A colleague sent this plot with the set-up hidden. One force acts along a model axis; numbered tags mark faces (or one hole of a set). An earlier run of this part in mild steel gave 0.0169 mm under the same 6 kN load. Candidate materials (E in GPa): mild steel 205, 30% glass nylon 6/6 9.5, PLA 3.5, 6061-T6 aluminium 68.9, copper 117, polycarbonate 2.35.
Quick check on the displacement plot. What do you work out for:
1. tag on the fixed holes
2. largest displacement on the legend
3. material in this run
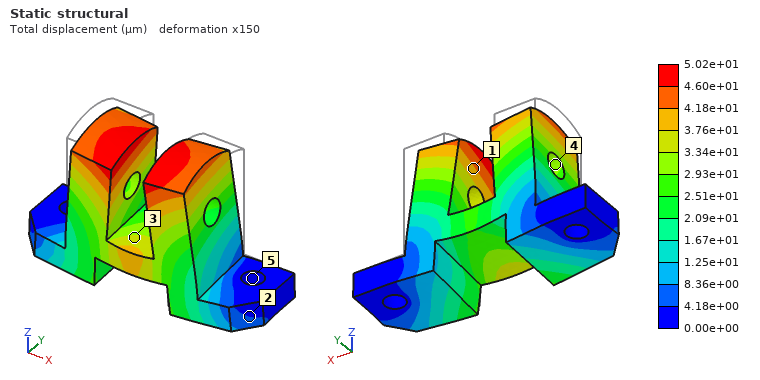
5
5.02e+01 µm
6061-T6 aluminium
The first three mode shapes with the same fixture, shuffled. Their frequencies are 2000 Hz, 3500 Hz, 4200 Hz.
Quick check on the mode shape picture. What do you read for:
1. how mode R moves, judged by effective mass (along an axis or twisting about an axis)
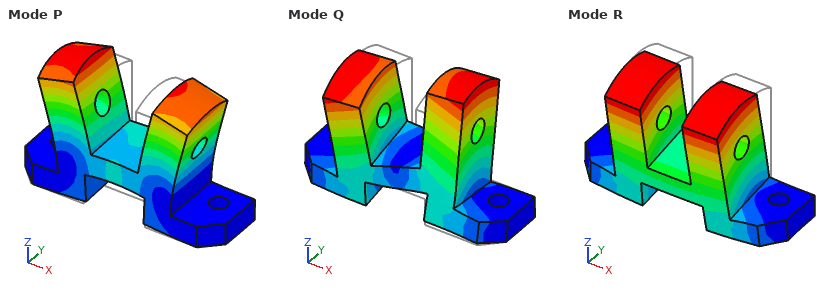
along Y
